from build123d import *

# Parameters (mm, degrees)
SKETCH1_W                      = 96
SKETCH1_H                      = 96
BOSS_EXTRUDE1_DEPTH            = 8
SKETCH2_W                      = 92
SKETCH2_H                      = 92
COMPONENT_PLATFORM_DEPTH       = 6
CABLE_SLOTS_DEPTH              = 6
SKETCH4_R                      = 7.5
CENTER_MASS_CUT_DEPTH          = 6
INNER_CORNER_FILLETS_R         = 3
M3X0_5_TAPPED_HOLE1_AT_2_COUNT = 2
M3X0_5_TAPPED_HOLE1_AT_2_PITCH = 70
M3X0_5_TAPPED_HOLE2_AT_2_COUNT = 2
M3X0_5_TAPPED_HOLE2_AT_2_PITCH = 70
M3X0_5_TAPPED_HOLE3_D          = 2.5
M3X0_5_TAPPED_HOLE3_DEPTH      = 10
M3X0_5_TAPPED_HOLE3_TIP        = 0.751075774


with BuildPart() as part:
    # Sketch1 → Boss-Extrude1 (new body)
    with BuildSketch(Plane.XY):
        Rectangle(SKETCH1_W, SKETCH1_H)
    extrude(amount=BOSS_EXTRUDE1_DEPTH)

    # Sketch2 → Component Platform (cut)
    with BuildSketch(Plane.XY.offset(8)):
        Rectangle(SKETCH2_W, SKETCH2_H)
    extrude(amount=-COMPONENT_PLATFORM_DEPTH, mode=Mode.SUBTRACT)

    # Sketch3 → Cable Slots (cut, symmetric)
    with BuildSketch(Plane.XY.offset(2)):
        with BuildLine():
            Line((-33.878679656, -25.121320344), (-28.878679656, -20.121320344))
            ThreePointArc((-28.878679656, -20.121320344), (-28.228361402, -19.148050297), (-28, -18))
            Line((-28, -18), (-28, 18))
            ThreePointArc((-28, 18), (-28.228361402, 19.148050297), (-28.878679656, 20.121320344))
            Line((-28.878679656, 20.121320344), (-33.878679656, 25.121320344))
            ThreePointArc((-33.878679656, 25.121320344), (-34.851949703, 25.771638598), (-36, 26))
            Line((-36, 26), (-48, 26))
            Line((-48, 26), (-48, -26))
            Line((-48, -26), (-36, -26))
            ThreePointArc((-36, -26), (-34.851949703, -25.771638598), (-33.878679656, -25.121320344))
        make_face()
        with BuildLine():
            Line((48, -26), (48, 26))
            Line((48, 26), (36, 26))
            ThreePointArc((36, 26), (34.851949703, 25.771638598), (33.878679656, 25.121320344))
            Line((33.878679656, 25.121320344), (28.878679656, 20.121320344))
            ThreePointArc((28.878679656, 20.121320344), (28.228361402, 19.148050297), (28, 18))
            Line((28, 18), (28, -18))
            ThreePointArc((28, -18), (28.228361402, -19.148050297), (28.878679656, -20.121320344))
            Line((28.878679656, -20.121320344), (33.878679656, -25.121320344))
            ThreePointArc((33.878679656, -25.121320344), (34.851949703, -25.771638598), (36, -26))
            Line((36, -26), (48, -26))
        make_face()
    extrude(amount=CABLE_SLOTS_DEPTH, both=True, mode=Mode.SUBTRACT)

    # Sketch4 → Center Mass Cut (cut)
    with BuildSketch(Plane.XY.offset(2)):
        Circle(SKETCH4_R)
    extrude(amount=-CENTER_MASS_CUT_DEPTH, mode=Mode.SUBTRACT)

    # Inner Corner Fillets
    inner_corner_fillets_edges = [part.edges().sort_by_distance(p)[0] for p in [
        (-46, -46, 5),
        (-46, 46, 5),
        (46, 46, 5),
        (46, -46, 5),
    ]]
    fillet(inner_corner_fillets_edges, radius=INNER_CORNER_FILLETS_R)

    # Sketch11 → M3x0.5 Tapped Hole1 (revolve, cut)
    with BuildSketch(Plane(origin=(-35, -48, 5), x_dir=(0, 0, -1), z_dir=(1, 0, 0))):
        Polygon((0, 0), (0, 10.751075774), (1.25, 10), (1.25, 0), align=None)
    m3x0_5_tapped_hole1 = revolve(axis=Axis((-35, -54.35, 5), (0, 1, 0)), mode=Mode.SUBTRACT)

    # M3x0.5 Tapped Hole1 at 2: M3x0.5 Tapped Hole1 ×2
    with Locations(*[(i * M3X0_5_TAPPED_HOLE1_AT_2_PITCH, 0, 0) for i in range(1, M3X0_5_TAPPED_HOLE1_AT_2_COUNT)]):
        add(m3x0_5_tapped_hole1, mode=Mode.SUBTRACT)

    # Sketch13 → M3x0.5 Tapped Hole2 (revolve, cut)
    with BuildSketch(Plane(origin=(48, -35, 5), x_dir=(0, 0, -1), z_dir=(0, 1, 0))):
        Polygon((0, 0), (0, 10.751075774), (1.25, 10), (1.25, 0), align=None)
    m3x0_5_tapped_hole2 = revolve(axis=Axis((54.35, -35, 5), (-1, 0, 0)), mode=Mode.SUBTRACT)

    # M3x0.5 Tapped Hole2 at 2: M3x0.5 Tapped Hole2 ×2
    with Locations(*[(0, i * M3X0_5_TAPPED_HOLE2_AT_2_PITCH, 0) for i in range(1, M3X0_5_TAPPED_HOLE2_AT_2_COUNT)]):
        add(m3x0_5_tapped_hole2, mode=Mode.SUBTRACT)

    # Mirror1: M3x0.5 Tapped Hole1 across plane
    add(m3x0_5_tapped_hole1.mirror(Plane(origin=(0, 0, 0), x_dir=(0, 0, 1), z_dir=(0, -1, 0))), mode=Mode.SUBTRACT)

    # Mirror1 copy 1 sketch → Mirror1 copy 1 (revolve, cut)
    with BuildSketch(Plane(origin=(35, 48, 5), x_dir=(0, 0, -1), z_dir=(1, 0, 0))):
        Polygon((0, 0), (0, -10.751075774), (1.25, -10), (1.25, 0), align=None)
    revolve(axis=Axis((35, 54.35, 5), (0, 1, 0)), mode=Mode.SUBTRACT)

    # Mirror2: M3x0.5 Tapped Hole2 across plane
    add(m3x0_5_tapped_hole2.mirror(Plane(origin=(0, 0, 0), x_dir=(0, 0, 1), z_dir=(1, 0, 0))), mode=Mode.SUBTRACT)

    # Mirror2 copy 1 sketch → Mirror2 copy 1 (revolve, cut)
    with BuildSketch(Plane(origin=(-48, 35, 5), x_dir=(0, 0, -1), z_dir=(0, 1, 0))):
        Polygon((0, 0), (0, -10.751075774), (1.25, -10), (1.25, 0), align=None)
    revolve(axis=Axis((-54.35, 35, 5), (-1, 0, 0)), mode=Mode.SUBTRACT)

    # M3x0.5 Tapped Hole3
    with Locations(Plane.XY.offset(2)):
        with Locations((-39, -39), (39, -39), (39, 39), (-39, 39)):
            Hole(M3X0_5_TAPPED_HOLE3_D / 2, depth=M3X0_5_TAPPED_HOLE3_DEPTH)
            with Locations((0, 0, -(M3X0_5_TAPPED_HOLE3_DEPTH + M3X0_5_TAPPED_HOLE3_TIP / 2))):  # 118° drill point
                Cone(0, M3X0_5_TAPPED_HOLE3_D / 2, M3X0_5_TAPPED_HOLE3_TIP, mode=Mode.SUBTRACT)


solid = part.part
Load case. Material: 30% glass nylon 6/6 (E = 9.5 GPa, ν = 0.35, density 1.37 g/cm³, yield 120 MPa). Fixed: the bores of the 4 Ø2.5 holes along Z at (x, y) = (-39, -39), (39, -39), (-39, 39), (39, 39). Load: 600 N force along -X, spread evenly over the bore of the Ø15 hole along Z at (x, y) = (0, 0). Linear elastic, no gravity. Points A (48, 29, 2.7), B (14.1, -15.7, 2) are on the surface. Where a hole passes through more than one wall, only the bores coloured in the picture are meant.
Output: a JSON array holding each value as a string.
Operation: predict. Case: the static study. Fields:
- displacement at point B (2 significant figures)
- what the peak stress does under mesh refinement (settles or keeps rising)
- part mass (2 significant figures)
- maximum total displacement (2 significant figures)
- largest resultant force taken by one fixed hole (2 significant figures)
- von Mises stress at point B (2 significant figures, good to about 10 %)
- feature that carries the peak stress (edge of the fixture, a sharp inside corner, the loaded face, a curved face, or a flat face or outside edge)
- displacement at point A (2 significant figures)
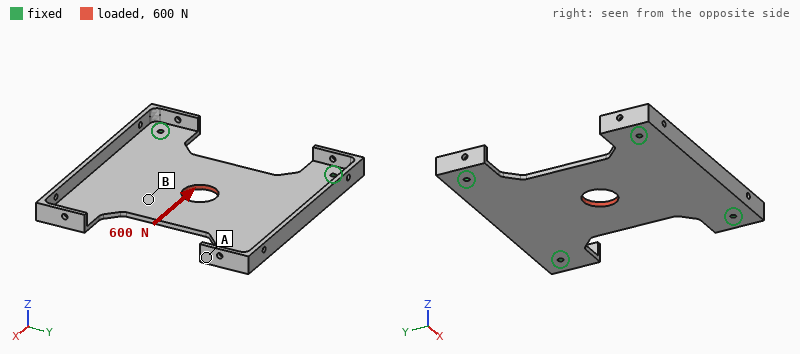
["23 µm", "keeps rising", "24 g", "38 µm", "180 N", "5.3 MPa", "edge of the fixture", "9.0 µm"]
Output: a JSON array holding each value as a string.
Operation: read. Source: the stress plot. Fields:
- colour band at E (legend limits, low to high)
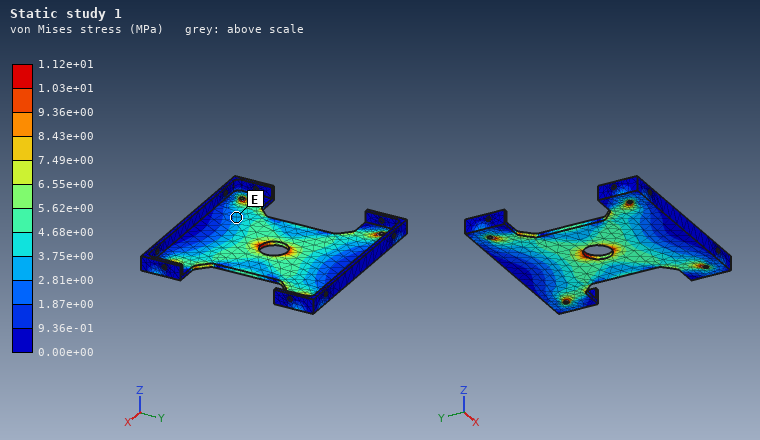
["2.81e+00 to 3.75e+00 MPa"]
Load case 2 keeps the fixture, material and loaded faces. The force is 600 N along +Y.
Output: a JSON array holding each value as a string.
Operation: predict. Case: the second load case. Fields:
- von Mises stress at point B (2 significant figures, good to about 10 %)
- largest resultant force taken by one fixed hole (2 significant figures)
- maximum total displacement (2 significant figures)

["5.0 MPa", "170 N", "57 µm"]
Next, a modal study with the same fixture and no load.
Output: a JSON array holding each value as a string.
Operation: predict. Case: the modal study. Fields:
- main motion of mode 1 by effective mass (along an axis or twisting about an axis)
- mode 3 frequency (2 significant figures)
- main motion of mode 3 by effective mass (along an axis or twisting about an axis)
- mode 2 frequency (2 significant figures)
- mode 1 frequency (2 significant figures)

["along Z", "1300 Hz", "twisting about X", "1200 Hz", "600 Hz"]
